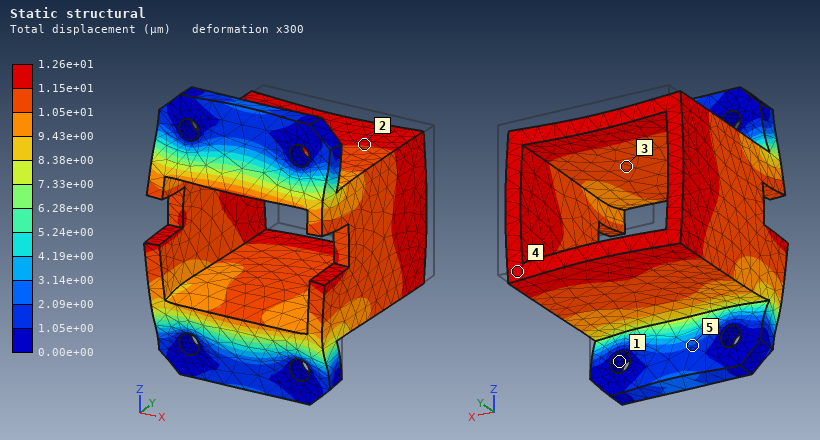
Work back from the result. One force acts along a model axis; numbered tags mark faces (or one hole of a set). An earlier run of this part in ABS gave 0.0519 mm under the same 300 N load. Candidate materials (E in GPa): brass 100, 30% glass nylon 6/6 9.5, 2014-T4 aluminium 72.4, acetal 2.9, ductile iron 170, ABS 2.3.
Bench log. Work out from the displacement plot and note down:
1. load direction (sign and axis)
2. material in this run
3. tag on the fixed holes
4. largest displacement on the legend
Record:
-Y
30% glass nylon 6/6
1
1.26e+01 µm
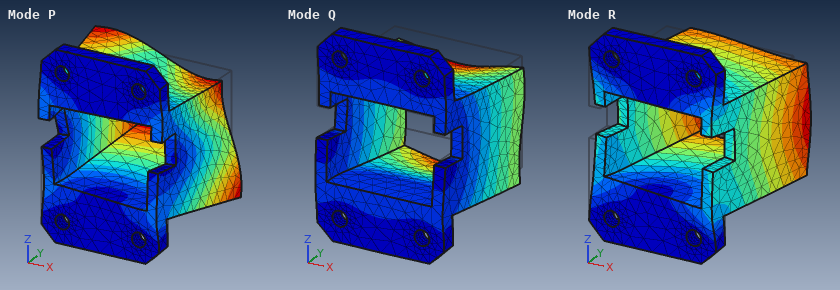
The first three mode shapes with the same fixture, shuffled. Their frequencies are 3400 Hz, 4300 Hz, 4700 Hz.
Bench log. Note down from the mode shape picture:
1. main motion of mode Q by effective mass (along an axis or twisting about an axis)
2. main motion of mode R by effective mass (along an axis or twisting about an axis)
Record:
along Z
along X
